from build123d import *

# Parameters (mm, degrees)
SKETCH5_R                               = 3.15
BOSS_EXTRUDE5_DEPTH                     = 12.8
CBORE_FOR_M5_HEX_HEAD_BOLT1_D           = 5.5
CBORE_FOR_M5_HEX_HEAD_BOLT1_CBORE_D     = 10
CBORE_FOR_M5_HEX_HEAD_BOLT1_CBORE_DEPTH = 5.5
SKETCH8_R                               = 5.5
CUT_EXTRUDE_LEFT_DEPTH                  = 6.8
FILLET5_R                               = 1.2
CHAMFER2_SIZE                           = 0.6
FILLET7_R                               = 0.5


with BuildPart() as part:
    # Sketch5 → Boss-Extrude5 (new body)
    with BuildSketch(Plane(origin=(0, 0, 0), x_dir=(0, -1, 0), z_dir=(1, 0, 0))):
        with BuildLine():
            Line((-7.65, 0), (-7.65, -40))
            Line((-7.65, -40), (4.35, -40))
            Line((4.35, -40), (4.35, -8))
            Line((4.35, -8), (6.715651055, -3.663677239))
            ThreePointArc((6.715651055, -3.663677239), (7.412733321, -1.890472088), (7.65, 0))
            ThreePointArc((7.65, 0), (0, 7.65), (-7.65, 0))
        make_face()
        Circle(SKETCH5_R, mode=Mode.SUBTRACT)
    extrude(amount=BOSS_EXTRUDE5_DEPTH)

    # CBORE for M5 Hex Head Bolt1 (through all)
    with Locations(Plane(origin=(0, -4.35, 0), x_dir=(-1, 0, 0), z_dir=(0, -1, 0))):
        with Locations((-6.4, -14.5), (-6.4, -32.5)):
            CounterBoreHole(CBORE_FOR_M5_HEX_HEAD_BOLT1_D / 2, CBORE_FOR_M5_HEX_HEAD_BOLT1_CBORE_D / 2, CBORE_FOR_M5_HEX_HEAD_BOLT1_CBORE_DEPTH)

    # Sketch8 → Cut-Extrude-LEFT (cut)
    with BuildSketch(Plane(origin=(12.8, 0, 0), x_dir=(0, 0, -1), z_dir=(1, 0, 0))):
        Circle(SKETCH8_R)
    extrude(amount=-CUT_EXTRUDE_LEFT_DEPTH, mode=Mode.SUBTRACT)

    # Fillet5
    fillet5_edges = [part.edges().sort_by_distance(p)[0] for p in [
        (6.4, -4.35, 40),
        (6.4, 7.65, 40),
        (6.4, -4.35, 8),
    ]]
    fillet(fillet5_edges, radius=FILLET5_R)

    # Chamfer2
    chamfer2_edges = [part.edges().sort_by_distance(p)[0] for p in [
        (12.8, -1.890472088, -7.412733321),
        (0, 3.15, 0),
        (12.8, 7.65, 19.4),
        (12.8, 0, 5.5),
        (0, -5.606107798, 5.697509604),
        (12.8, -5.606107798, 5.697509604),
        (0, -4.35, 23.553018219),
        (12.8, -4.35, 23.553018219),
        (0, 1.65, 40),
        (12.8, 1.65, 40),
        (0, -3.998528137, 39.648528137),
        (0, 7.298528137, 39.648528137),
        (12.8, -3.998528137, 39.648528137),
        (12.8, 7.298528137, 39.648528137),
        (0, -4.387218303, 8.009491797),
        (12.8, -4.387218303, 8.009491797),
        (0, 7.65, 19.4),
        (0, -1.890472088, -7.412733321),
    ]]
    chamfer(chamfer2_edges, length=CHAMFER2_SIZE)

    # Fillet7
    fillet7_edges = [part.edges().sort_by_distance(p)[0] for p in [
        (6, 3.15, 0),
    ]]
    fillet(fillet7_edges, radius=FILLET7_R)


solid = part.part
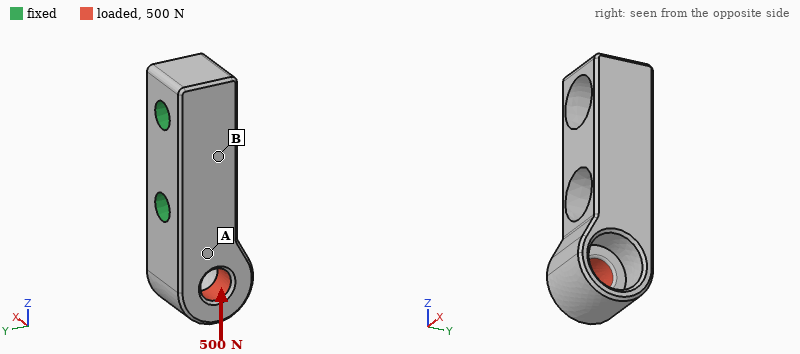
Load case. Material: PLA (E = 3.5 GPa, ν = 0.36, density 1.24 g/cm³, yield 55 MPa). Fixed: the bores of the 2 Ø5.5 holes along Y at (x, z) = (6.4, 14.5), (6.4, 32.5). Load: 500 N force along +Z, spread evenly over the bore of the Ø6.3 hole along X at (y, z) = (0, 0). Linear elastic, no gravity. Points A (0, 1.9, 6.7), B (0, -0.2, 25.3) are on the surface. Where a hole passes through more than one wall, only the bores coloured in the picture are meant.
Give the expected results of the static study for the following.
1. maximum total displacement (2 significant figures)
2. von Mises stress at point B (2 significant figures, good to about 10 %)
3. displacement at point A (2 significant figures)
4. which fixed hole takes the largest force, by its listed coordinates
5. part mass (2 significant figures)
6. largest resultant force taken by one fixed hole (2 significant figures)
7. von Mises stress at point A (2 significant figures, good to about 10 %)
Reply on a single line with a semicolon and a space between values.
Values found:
0.17 mm; 3.4 MPa; 0.049 mm; (6.4, 14.5); 6.8 g; 410 N; 9.4 MPa
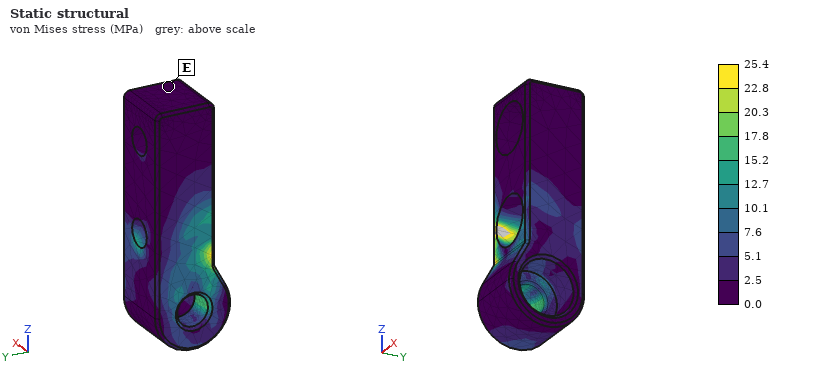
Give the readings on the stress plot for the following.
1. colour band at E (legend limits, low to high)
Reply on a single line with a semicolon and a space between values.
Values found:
0.0 to 2.5 MPa
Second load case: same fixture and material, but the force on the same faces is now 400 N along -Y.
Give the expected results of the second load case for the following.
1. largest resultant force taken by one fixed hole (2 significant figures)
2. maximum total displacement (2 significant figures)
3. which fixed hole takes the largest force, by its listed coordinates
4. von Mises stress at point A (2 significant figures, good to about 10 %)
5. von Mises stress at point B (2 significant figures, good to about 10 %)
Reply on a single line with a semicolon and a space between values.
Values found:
520 N; 0.38 mm; (6.4, 14.5); 16 MPa; 3.9 MPa
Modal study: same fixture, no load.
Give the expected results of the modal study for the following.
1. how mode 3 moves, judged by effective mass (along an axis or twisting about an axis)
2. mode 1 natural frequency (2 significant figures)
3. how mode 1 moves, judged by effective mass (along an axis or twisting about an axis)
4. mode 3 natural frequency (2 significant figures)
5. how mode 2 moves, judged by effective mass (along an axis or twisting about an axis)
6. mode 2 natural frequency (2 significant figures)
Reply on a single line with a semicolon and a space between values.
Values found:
twisting about Z; 4200 Hz; along Y; 8500 Hz; along X; 5000 Hz
